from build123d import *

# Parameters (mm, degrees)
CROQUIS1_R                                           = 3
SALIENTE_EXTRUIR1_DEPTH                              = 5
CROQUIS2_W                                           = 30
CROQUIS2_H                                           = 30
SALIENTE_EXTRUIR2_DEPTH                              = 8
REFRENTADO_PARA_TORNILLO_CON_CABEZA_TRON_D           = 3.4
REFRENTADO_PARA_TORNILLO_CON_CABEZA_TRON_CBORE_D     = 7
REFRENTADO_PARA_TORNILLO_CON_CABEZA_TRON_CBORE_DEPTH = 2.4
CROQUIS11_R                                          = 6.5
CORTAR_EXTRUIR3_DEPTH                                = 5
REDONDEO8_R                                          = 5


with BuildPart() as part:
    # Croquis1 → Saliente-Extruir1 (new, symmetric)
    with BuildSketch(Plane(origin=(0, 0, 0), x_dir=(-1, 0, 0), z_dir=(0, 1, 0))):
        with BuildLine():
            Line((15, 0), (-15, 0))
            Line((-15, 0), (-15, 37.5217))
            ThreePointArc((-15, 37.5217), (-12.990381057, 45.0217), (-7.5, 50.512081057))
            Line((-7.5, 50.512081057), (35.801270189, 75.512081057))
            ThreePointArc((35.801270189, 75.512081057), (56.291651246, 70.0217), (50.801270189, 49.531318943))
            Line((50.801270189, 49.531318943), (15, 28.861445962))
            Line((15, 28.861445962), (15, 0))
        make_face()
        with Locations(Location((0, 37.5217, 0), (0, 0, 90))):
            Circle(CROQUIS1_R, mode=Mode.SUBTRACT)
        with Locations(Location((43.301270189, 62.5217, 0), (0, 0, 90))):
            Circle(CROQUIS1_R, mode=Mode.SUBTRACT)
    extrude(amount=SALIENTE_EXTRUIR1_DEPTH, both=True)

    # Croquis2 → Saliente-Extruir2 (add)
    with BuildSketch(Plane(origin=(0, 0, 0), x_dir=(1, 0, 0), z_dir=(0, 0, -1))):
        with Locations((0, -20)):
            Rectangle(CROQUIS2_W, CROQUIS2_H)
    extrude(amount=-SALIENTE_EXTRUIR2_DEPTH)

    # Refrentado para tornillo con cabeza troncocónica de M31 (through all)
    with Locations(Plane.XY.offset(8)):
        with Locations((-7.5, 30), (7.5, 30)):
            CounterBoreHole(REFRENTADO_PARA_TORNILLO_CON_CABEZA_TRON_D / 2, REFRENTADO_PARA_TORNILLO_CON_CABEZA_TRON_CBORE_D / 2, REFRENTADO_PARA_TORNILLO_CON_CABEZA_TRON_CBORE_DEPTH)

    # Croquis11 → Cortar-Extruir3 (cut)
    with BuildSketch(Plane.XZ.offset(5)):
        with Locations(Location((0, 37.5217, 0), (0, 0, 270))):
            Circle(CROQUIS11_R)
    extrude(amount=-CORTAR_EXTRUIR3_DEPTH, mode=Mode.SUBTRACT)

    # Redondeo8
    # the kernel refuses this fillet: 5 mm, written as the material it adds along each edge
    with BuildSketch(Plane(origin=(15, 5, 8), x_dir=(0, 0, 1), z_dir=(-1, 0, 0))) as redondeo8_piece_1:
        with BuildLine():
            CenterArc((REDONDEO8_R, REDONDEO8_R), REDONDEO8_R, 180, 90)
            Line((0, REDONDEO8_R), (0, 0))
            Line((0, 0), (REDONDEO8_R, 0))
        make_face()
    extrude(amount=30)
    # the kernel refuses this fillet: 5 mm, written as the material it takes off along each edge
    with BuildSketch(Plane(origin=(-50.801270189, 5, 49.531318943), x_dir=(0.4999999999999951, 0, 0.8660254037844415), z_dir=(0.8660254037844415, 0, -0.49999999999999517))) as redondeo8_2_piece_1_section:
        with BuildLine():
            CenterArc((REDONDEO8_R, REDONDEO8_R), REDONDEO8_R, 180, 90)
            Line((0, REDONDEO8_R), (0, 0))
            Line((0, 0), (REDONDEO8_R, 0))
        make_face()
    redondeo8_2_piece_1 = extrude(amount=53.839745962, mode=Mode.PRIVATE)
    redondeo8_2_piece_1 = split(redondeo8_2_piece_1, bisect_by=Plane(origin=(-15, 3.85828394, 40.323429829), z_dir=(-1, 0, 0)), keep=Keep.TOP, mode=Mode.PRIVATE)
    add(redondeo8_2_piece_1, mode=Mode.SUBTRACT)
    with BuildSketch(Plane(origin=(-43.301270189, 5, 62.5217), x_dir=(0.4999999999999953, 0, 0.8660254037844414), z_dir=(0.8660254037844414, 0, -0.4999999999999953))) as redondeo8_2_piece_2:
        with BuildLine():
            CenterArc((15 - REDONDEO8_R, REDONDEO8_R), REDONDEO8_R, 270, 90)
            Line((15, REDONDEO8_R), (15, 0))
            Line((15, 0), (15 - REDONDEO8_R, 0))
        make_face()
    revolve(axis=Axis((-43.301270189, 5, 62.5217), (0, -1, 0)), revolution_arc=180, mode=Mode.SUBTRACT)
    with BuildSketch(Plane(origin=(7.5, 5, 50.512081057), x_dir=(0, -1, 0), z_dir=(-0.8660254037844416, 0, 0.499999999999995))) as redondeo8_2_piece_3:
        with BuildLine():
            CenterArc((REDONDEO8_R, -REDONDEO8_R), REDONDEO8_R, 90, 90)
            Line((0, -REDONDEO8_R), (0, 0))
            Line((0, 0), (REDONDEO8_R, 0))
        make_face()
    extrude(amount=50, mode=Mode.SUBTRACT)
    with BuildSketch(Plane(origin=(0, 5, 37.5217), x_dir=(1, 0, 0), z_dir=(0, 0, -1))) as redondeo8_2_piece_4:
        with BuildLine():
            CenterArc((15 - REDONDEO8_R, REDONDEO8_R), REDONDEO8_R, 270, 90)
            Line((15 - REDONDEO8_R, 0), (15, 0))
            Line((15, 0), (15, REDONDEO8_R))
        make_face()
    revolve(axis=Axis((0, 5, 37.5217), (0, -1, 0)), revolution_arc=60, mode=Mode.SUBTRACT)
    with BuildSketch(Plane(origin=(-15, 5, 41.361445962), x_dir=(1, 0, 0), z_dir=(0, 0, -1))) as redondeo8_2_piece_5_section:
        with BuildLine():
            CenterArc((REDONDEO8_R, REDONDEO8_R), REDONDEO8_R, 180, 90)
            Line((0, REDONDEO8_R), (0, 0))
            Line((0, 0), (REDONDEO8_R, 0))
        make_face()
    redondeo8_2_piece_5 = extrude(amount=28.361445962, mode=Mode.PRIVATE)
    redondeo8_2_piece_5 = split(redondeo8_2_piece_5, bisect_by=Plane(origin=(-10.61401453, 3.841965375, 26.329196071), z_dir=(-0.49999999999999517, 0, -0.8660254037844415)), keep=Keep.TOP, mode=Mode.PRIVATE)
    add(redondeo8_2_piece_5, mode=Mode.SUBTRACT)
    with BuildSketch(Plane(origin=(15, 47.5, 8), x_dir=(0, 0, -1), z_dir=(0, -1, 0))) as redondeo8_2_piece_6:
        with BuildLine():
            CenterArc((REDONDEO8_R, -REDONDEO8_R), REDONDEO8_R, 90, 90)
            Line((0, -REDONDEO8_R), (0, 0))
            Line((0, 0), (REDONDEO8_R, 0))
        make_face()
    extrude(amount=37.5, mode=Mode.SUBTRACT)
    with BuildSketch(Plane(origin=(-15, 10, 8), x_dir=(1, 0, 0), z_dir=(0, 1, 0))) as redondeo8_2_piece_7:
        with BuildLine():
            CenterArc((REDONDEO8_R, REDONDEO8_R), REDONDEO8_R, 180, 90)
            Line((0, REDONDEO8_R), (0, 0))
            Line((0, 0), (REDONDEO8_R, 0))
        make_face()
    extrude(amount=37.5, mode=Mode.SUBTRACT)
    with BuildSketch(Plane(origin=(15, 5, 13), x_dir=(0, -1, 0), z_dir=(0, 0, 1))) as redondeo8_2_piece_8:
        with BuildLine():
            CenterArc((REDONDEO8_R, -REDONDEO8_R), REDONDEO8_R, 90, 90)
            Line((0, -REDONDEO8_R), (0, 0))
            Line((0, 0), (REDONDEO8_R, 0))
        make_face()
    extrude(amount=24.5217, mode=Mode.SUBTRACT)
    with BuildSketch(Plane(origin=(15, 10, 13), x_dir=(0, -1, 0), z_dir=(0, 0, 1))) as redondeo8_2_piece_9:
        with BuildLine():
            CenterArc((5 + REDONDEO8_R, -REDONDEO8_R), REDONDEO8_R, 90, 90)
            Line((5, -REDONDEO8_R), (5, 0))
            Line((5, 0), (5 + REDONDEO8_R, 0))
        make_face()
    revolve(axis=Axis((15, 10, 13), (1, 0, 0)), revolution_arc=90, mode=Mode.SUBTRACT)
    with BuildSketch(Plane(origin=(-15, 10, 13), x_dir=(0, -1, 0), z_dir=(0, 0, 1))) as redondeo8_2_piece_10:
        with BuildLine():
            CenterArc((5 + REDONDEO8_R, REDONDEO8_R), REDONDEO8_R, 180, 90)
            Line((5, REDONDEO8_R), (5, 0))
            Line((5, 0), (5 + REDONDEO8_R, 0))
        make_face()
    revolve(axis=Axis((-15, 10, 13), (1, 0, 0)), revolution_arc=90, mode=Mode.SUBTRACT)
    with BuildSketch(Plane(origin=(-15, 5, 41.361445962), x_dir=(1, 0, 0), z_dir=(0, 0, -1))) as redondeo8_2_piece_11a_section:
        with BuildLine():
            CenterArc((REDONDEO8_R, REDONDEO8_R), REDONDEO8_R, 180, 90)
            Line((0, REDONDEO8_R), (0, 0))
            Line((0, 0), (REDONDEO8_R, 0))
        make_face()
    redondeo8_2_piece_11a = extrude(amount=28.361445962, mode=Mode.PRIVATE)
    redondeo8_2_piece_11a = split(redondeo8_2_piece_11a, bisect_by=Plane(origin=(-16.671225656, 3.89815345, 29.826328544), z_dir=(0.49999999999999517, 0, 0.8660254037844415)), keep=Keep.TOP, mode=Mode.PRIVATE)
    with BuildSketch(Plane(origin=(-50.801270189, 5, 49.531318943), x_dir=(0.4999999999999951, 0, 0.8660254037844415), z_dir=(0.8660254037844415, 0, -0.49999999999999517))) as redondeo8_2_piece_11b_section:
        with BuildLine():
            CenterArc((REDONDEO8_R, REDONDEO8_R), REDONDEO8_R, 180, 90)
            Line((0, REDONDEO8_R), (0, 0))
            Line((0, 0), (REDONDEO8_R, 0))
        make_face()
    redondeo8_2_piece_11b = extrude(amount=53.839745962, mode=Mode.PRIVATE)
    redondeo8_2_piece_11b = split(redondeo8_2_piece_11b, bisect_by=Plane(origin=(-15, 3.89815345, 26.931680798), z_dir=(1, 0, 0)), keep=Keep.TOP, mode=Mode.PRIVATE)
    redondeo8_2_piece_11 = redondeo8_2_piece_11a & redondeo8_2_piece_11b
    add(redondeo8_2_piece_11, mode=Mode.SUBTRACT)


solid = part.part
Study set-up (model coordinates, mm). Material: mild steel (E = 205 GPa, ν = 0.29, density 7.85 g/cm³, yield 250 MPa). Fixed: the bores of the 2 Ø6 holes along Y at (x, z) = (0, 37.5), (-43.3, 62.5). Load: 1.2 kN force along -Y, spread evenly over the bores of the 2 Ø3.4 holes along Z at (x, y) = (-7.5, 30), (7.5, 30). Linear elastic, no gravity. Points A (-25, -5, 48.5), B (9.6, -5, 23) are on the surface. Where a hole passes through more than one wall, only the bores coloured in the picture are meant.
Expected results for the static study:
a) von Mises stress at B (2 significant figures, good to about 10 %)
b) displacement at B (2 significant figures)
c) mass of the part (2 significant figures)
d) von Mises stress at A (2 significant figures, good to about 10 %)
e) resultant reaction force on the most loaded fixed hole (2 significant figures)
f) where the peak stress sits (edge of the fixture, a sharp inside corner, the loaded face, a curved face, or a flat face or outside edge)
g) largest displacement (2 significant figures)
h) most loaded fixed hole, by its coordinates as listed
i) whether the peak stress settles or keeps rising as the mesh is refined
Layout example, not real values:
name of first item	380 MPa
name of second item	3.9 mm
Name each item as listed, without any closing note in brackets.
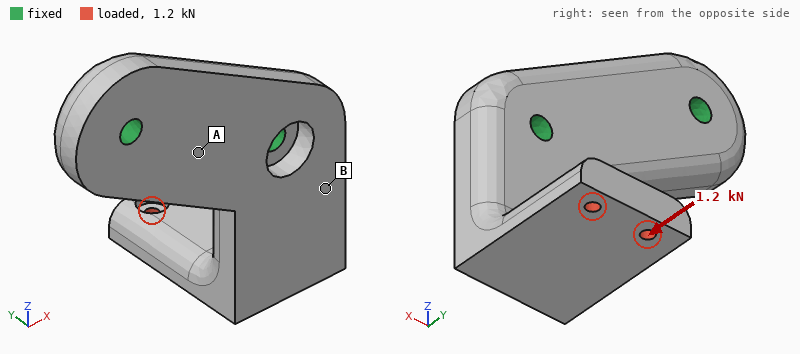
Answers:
von Mises stress at B	50 MPa
displacement at B	0.025 mm
mass of the part	270 g
von Mises stress at A	25 MPa
resultant reaction force on the most loaded fixed hole	1.6 kN
where the peak stress sits	edge of the fixture
largest displacement	0.12 mm
most loaded fixed hole, by its coordinates as listed	(0, 37.5)
whether the peak stress settles or keeps rising as the mesh is refined	keeps rising
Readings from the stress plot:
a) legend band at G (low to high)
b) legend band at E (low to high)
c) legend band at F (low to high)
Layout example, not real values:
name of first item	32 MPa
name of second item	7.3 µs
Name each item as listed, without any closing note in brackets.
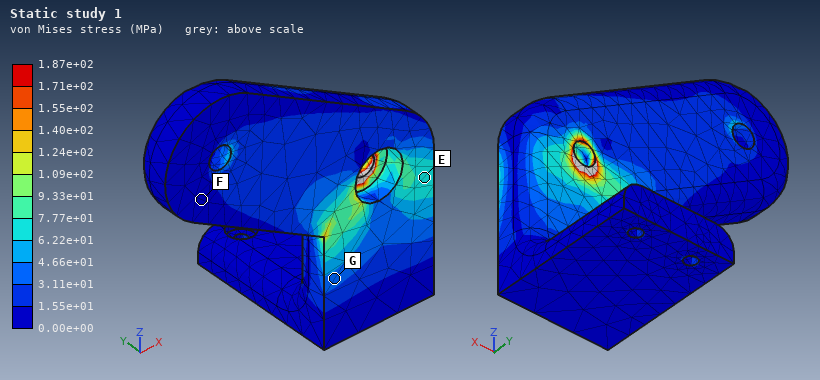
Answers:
legend band at G	3.11e+01 to 4.66e+01 MPa
legend band at E	6.22e+01 to 7.77e+01 MPa
legend band at F	0.00e+00 to 1.55e+01 MPa
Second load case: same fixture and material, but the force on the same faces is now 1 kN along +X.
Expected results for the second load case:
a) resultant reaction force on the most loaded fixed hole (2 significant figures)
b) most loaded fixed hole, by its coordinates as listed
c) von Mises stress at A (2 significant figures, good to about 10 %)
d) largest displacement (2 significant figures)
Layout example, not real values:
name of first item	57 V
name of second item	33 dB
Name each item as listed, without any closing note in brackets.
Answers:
resultant reaction force on the most loaded fixed hole	1.7 kN
most loaded fixed hole, by its coordinates as listed	(0, 37.5)
von Mises stress at A	19 MPa
largest displacement	79 µm
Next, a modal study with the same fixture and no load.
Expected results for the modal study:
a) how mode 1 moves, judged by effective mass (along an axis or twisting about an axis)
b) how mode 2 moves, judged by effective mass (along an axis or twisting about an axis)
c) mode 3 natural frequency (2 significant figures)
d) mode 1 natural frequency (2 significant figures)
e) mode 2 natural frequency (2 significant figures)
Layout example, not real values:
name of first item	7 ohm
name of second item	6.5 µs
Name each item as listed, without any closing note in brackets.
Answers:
how mode 1 moves, judged by effective mass	along Y
how mode 2 moves, judged by effective mass	along X
mode 3 natural frequency	5900 Hz
mode 1 natural frequency	2000 Hz
mode 2 natural frequency	3400 Hz
